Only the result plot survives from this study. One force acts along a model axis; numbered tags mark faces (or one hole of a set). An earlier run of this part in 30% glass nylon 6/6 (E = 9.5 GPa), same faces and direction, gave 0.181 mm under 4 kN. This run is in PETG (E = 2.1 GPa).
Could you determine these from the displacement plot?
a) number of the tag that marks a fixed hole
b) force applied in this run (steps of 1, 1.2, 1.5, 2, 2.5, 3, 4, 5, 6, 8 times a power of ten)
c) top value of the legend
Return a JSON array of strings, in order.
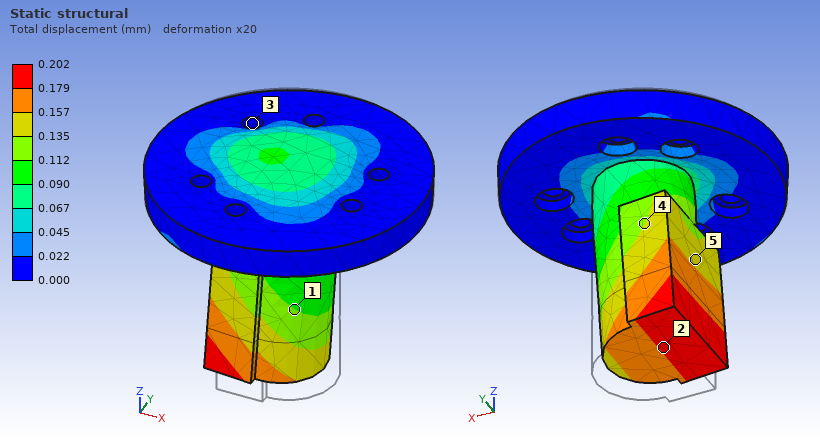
["3", "1 kN", "0.202 mm"]
